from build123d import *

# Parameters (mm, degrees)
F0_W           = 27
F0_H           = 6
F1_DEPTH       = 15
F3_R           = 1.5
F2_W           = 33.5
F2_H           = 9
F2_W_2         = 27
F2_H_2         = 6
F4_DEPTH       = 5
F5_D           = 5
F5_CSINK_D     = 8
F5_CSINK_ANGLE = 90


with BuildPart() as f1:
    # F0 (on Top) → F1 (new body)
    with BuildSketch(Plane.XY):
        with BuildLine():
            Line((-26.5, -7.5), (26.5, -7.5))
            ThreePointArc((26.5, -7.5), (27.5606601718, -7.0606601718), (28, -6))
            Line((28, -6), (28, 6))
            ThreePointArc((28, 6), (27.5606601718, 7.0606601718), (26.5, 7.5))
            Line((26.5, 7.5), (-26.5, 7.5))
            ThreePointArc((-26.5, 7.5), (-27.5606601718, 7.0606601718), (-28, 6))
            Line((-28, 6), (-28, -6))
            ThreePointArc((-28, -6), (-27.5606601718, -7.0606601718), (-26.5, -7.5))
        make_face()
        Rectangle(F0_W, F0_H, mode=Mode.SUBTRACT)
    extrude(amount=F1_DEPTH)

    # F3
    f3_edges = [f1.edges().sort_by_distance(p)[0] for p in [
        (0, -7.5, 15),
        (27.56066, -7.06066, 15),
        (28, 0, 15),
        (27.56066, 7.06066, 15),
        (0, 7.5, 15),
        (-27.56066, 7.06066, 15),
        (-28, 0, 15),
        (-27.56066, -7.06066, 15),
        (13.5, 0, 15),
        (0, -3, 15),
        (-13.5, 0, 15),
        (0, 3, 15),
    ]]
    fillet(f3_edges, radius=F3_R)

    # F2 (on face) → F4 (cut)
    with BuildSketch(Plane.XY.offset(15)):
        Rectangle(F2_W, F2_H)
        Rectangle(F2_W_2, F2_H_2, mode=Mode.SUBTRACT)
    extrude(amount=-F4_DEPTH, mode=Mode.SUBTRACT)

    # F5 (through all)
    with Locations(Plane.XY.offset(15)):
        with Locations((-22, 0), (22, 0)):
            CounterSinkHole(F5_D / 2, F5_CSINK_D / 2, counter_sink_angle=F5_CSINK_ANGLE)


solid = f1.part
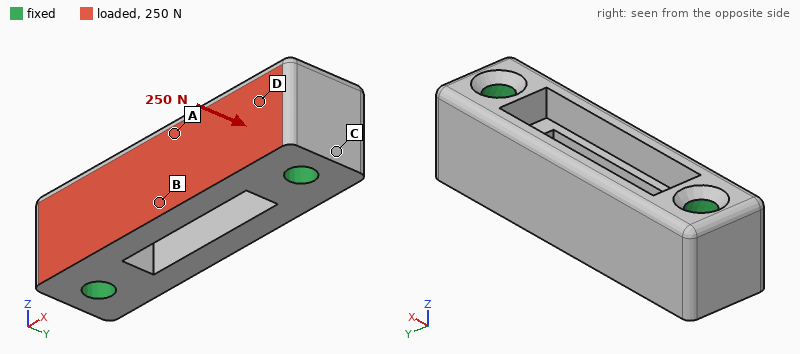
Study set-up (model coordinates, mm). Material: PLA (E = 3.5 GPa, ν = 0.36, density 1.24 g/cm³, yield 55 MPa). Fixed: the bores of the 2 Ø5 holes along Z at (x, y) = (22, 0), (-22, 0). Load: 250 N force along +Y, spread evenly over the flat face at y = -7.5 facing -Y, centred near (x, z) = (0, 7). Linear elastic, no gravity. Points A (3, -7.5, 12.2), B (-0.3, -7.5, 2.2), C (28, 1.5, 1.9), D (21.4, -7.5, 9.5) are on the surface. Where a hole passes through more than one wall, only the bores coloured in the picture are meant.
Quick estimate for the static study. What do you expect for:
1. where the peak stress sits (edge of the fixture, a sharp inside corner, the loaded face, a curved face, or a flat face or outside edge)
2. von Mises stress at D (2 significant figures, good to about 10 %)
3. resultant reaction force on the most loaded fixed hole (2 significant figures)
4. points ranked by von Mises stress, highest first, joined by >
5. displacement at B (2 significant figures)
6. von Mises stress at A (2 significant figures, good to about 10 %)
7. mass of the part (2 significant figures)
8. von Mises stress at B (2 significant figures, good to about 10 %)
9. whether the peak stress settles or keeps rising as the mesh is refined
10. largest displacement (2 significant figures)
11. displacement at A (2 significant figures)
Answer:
a sharp inside corner
1.3 MPa
130 N
B > A > D > C
49 µm
4.6 MPa
11 g
5.6 MPa
keeps rising
72 µm
61 µm
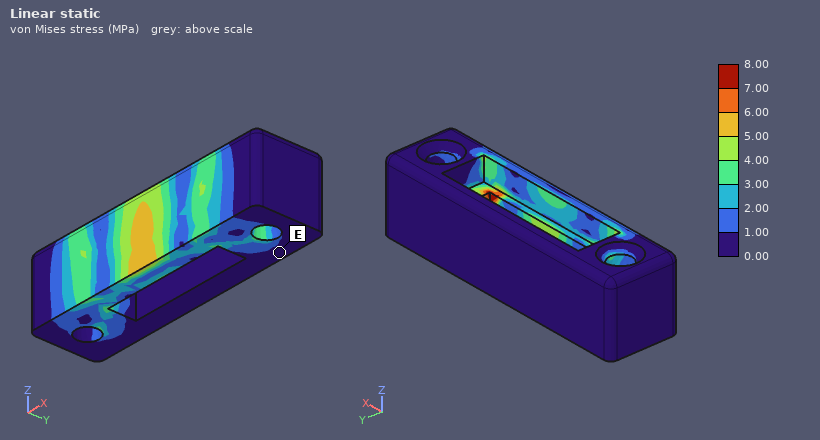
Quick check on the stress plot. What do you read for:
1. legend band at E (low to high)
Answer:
0.00 to 1.00 MPa
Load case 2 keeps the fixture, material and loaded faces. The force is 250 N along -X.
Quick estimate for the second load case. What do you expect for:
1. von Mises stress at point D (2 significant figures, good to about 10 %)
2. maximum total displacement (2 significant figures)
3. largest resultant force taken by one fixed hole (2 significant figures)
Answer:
0.79 MPa
8.5 µm
130 N
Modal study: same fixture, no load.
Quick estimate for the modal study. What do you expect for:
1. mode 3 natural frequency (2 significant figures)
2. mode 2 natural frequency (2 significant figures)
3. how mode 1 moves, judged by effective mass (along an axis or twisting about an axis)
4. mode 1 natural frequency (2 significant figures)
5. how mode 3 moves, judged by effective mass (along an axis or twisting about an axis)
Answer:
9000 Hz
6300 Hz
along Y
5700 Hz
twisting about X
